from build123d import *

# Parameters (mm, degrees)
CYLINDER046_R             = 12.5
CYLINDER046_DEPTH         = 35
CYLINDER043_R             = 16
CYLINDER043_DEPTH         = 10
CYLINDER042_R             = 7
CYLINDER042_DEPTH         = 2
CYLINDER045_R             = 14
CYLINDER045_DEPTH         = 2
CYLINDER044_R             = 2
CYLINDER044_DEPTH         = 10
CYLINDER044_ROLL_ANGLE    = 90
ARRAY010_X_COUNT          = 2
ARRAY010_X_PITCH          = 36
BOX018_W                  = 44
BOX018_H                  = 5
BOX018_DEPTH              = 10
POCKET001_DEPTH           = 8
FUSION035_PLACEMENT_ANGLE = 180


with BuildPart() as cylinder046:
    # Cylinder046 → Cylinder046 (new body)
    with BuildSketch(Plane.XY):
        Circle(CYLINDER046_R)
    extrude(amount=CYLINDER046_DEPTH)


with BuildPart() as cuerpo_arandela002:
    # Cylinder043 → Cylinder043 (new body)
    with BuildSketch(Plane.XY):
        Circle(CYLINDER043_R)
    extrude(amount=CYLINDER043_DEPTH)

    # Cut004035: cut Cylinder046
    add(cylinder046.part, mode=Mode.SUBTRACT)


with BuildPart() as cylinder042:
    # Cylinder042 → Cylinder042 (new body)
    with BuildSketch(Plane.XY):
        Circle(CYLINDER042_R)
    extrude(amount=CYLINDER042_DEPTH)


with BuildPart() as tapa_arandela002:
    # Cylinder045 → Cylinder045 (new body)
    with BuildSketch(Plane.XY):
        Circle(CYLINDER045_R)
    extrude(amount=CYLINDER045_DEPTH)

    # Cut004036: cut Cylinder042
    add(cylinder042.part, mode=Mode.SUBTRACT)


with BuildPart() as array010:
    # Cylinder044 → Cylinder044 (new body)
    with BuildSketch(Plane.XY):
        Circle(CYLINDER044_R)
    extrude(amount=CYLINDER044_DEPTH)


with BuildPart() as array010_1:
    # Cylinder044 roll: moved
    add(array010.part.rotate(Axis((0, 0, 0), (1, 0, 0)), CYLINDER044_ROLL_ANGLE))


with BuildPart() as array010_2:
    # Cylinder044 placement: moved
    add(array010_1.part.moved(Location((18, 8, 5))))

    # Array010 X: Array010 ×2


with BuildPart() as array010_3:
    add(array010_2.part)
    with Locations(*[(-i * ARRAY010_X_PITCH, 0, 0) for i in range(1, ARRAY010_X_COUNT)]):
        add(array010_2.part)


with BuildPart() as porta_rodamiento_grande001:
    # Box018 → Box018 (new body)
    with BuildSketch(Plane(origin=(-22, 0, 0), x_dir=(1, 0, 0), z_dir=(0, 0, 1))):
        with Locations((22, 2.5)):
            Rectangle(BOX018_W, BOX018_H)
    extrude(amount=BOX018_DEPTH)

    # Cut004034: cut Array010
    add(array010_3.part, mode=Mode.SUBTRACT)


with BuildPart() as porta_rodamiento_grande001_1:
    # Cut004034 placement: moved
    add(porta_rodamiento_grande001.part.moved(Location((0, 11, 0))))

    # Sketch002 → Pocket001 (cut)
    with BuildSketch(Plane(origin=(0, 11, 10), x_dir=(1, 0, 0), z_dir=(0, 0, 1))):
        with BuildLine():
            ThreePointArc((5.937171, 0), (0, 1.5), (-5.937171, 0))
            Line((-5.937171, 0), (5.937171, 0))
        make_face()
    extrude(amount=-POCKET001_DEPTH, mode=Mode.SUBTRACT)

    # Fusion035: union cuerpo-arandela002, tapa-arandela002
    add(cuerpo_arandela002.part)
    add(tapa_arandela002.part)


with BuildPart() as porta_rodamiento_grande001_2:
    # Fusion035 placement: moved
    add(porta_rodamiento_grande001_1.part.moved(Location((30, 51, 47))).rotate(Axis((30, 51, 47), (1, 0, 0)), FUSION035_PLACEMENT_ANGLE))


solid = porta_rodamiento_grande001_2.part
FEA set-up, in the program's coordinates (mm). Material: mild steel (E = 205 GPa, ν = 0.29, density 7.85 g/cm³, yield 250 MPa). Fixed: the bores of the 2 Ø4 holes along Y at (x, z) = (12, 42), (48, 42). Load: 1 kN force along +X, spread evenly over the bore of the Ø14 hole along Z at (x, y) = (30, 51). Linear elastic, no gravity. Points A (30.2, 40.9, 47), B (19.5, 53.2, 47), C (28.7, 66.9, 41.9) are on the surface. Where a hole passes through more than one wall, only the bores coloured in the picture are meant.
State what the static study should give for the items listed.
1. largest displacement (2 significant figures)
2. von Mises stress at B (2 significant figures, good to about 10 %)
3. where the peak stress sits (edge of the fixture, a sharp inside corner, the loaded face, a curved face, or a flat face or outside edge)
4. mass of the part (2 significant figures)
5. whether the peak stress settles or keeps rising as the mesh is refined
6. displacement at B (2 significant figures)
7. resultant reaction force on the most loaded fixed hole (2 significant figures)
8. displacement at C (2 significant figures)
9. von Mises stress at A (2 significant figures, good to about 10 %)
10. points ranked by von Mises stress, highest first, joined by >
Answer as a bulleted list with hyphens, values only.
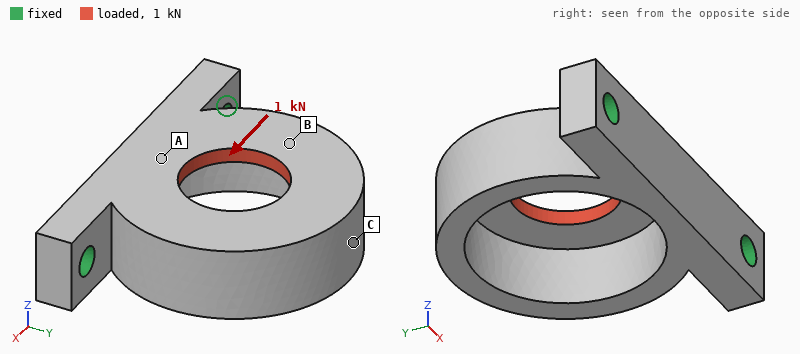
- 17 µm
- 22 MPa
- edge of the fixture
- 40 g
- keeps rising
- 11 µm
- 700 N
- 16 µm
- 38 MPa
- A > B > C
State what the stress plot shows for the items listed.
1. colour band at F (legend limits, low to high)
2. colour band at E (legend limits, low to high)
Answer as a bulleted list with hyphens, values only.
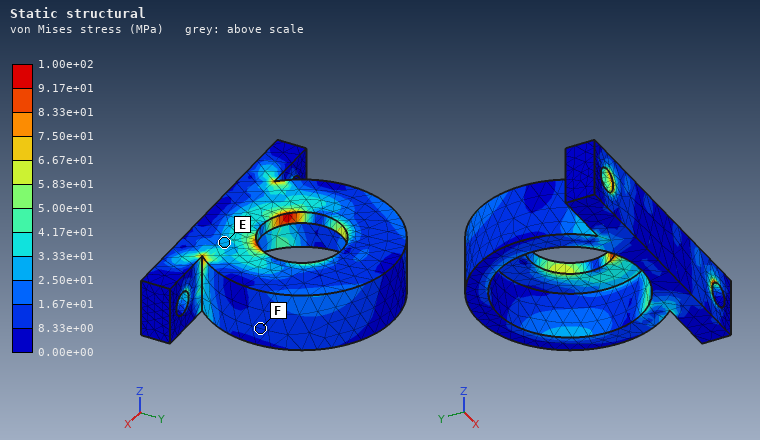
- 8.33e+00 to 1.67e+01 MPa
- 2.50e+01 to 3.33e+01 MPa
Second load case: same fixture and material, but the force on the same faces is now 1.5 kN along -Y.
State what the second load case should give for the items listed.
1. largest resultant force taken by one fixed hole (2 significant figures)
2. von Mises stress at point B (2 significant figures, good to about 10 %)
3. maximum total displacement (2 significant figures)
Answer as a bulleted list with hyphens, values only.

- 760 N
- 20 MPa
- 33 µm
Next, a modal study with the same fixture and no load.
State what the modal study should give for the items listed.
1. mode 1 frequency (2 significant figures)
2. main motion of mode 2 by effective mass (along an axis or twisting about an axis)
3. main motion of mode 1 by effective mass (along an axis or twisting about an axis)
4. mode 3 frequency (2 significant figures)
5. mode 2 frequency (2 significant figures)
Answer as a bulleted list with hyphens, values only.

- 3900 Hz
- along X
- along Z
- 13 kHz
- 7000 Hz
